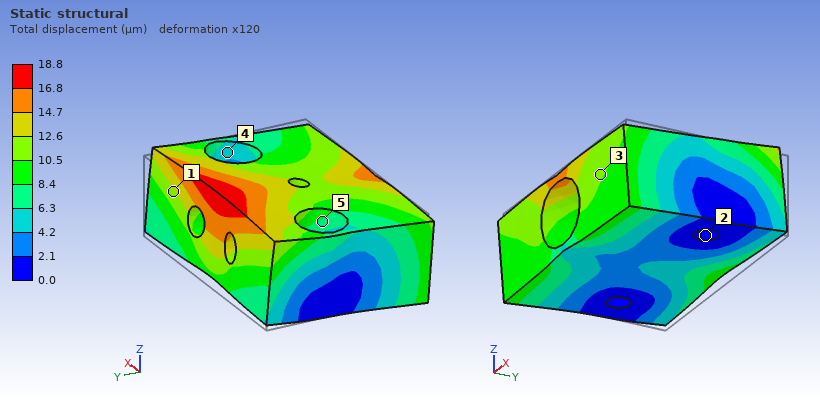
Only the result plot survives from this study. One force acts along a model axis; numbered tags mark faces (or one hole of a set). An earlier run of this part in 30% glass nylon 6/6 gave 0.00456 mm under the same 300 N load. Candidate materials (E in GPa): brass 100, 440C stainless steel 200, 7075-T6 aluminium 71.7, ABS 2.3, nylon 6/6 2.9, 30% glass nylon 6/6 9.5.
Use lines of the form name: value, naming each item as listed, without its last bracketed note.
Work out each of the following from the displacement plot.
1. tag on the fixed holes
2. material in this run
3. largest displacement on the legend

tag on the fixed holes: 2
material in this run: ABS
largest displacement on the legend: 18.8 µm
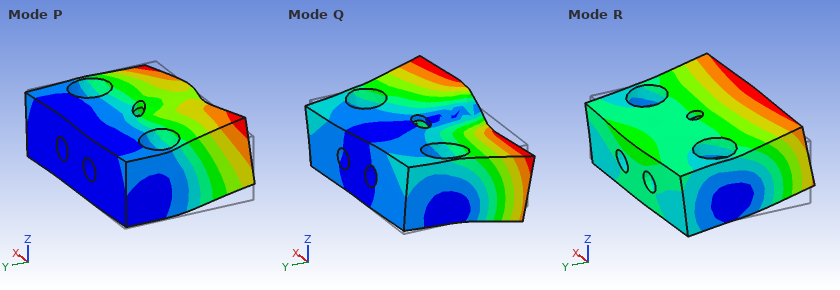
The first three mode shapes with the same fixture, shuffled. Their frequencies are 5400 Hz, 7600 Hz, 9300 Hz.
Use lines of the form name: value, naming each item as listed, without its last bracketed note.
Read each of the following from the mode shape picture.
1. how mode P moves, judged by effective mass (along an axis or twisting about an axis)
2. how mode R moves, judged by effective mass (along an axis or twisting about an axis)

how mode P moves, judged by effective mass: along X
how mode R moves, judged by effective mass: along Z
